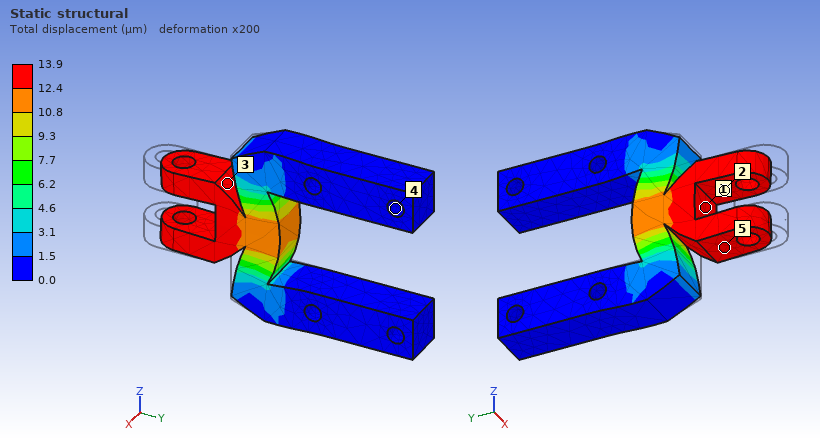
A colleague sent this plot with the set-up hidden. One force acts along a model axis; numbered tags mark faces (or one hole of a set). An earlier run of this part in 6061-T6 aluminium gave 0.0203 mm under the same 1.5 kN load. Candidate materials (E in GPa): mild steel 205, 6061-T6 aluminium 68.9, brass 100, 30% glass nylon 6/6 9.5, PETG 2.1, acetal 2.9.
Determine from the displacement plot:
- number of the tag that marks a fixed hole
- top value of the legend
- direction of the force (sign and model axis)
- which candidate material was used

4
13.9 µm
+Y
brass
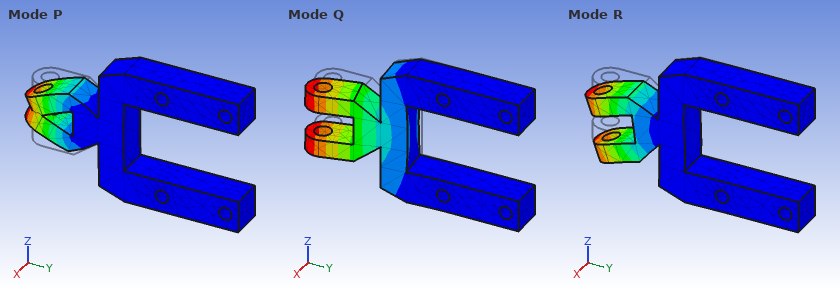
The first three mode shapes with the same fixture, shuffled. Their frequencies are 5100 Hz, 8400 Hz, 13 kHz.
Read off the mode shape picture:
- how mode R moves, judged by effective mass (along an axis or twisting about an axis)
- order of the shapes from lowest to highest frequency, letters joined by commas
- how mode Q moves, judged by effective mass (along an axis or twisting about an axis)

along Z
Q, R, P
along X
